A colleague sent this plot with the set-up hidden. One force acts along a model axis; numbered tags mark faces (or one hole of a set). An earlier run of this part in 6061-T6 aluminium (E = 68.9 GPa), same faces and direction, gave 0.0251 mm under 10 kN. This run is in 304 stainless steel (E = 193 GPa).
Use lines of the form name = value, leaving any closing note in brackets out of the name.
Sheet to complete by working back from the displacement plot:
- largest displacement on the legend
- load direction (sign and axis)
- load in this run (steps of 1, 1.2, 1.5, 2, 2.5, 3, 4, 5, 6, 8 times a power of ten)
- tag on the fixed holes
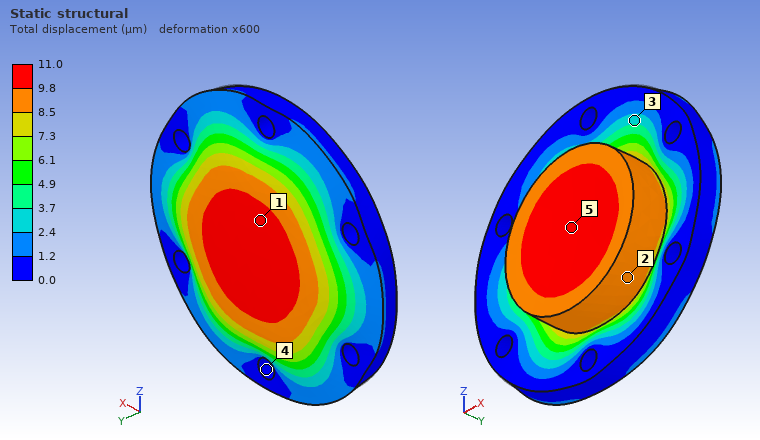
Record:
largest displacement on the legend = 11.0 µm
load direction = +Y
load in this run = 12 kN
tag on the fixed holes = 4
